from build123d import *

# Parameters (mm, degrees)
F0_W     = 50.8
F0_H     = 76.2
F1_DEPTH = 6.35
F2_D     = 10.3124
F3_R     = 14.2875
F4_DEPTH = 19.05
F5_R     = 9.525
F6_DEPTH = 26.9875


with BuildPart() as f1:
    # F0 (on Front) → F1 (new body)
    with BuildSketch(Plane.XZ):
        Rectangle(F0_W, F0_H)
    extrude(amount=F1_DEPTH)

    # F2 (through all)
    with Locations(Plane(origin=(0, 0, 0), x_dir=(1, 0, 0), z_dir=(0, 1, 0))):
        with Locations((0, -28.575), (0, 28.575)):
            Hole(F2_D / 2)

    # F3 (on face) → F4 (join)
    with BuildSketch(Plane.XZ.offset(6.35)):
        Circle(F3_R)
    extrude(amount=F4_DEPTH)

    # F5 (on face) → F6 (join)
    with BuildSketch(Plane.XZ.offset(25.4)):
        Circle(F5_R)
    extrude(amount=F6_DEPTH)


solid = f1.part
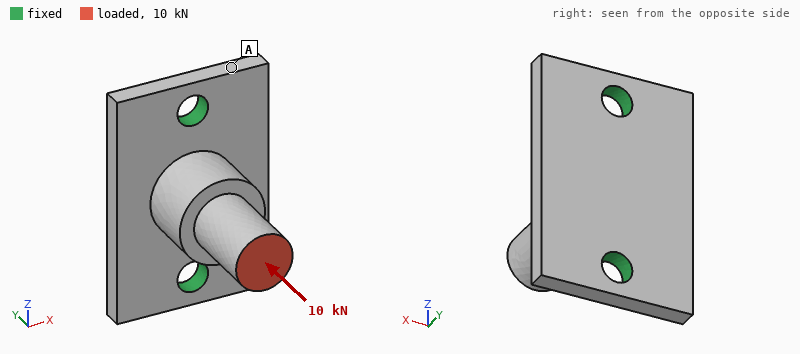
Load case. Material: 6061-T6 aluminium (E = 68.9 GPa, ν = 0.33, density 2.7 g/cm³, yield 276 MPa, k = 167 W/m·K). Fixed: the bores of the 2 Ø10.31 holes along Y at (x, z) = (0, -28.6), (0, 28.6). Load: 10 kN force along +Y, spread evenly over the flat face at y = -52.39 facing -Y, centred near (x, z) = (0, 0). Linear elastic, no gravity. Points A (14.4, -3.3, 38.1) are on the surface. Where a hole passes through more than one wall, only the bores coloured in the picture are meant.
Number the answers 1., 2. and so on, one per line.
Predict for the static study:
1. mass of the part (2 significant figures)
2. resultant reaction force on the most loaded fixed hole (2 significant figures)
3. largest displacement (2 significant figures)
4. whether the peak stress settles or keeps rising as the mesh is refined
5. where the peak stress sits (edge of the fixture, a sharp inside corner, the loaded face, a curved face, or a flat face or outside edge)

1. 120 g
2. 5.3 kN
3. 76 µm
4. keeps rising
5. edge of the fixture
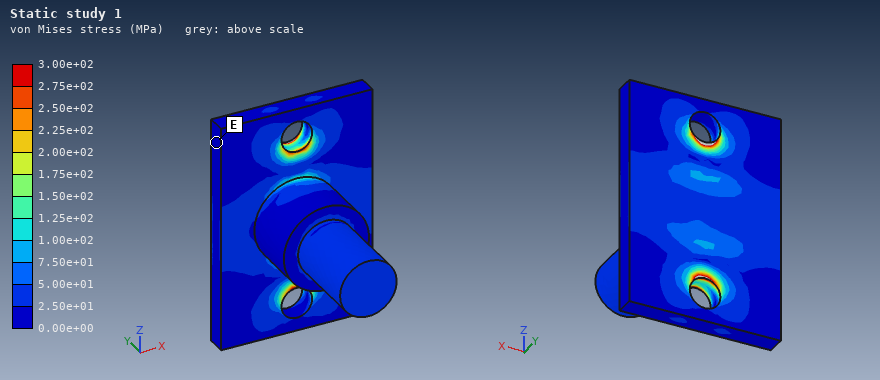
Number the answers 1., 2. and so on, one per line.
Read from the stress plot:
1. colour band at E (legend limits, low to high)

1. 0.00e+00 to 2.50e+01 MPa
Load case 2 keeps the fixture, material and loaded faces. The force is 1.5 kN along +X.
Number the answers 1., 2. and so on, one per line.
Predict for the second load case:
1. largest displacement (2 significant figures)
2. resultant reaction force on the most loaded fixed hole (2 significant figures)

1. 0.31 mm
2. 750 N
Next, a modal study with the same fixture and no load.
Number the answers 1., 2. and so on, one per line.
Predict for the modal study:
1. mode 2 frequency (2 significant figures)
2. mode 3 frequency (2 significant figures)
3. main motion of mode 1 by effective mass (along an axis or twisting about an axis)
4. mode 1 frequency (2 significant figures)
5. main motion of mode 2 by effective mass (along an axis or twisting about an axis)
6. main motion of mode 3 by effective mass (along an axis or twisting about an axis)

1. 5700 Hz
2. 7100 Hz
3. along X
4. 2800 Hz
5. along Z
6. along Y
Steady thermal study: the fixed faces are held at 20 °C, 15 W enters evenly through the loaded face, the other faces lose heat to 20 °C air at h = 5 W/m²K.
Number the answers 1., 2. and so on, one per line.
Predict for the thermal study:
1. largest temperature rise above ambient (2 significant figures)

1. 15 K
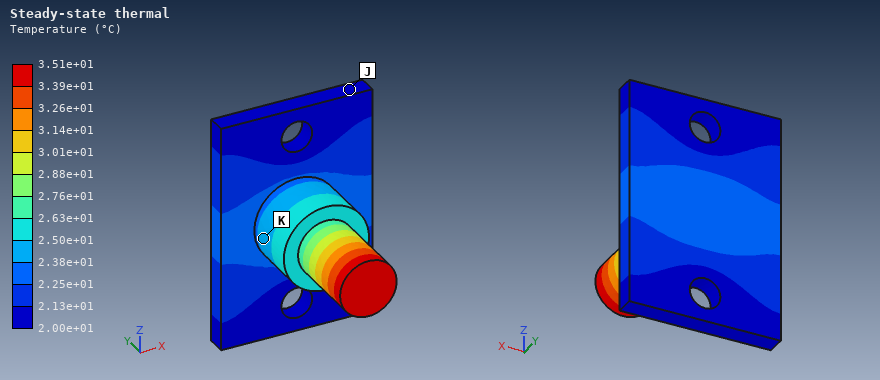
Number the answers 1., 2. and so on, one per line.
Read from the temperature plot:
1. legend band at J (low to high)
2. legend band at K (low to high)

1. 2.00e+01 to 2.13e+01 °C
2. 2.38e+01 to 2.50e+01 °C
